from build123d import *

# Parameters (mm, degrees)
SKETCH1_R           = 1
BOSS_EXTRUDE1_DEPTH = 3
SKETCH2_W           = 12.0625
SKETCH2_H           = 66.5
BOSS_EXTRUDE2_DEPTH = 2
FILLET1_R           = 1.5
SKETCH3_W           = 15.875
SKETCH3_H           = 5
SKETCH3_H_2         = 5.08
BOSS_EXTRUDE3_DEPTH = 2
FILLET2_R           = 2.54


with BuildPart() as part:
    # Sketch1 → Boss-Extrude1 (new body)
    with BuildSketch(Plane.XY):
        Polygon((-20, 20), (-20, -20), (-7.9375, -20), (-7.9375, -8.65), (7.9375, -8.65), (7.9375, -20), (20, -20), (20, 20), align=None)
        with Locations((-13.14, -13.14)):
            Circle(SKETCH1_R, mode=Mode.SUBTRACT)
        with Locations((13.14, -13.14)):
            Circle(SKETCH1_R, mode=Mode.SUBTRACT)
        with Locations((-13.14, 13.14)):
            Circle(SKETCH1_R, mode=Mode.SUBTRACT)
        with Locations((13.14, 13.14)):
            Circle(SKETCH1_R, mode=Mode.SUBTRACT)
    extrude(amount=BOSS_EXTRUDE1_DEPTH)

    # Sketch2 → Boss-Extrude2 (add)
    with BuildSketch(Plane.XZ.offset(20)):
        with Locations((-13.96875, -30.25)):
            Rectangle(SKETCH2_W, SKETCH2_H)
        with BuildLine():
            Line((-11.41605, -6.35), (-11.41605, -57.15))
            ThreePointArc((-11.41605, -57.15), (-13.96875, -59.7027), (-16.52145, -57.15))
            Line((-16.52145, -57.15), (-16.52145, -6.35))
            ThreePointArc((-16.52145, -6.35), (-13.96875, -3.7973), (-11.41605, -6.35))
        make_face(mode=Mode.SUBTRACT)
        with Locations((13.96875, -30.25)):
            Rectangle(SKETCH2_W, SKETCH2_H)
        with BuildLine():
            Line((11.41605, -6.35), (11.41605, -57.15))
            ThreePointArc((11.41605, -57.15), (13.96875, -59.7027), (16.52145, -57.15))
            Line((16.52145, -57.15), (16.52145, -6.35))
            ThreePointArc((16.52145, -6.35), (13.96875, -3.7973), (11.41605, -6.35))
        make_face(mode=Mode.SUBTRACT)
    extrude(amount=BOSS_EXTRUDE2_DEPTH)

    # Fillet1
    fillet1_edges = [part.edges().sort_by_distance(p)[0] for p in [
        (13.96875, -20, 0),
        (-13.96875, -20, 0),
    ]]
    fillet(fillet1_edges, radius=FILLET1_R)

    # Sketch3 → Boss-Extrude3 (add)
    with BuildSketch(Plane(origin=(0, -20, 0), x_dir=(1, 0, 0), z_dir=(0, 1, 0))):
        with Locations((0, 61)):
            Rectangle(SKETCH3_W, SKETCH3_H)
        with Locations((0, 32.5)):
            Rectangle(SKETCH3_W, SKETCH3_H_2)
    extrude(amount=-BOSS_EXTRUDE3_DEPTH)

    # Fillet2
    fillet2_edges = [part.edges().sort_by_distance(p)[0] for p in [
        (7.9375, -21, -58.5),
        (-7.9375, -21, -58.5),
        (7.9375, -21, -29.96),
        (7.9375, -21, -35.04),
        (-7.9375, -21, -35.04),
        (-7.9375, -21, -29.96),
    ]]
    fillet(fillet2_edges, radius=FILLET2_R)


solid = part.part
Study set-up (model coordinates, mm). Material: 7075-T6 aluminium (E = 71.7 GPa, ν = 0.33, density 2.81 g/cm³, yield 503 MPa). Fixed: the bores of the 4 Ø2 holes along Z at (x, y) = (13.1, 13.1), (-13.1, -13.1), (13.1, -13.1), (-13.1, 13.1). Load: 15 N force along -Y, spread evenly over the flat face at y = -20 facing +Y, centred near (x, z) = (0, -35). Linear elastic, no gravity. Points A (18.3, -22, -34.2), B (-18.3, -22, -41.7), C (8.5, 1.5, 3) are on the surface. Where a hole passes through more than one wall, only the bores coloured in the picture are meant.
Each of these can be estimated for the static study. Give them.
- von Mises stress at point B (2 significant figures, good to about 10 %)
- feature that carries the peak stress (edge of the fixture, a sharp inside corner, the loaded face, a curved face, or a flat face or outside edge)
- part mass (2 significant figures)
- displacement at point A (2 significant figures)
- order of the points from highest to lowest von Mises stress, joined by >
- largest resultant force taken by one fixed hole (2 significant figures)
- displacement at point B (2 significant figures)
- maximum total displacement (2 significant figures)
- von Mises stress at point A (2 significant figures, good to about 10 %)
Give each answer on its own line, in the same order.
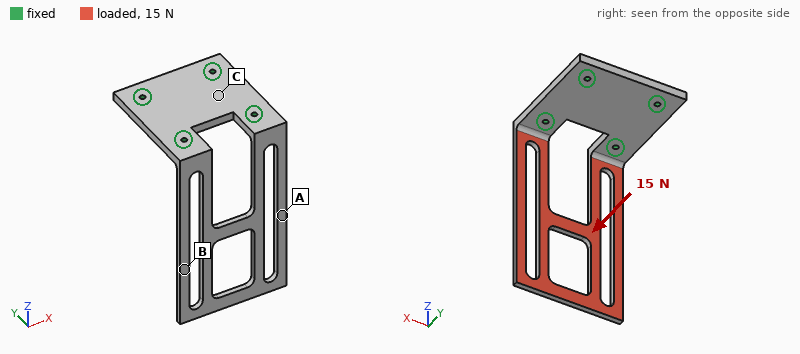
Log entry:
8.6 MPa
the loaded face
19 g
0.32 mm
A > B > C
7.4 N
0.45 mm
0.83 mm
14 MPa
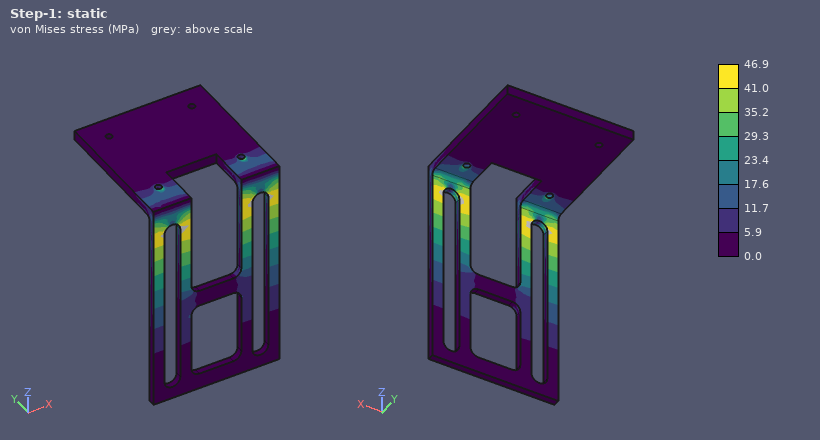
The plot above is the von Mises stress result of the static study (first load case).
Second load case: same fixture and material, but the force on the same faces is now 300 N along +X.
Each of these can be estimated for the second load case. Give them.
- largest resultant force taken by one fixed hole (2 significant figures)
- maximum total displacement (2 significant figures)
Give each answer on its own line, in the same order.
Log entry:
370 N
0.78 mm
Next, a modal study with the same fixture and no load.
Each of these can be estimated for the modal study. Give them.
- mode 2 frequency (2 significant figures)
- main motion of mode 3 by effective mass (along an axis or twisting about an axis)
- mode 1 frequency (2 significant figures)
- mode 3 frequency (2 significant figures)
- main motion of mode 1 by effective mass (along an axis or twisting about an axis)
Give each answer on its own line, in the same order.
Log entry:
1000 Hz
along X
330 Hz
1500 Hz
along Y
